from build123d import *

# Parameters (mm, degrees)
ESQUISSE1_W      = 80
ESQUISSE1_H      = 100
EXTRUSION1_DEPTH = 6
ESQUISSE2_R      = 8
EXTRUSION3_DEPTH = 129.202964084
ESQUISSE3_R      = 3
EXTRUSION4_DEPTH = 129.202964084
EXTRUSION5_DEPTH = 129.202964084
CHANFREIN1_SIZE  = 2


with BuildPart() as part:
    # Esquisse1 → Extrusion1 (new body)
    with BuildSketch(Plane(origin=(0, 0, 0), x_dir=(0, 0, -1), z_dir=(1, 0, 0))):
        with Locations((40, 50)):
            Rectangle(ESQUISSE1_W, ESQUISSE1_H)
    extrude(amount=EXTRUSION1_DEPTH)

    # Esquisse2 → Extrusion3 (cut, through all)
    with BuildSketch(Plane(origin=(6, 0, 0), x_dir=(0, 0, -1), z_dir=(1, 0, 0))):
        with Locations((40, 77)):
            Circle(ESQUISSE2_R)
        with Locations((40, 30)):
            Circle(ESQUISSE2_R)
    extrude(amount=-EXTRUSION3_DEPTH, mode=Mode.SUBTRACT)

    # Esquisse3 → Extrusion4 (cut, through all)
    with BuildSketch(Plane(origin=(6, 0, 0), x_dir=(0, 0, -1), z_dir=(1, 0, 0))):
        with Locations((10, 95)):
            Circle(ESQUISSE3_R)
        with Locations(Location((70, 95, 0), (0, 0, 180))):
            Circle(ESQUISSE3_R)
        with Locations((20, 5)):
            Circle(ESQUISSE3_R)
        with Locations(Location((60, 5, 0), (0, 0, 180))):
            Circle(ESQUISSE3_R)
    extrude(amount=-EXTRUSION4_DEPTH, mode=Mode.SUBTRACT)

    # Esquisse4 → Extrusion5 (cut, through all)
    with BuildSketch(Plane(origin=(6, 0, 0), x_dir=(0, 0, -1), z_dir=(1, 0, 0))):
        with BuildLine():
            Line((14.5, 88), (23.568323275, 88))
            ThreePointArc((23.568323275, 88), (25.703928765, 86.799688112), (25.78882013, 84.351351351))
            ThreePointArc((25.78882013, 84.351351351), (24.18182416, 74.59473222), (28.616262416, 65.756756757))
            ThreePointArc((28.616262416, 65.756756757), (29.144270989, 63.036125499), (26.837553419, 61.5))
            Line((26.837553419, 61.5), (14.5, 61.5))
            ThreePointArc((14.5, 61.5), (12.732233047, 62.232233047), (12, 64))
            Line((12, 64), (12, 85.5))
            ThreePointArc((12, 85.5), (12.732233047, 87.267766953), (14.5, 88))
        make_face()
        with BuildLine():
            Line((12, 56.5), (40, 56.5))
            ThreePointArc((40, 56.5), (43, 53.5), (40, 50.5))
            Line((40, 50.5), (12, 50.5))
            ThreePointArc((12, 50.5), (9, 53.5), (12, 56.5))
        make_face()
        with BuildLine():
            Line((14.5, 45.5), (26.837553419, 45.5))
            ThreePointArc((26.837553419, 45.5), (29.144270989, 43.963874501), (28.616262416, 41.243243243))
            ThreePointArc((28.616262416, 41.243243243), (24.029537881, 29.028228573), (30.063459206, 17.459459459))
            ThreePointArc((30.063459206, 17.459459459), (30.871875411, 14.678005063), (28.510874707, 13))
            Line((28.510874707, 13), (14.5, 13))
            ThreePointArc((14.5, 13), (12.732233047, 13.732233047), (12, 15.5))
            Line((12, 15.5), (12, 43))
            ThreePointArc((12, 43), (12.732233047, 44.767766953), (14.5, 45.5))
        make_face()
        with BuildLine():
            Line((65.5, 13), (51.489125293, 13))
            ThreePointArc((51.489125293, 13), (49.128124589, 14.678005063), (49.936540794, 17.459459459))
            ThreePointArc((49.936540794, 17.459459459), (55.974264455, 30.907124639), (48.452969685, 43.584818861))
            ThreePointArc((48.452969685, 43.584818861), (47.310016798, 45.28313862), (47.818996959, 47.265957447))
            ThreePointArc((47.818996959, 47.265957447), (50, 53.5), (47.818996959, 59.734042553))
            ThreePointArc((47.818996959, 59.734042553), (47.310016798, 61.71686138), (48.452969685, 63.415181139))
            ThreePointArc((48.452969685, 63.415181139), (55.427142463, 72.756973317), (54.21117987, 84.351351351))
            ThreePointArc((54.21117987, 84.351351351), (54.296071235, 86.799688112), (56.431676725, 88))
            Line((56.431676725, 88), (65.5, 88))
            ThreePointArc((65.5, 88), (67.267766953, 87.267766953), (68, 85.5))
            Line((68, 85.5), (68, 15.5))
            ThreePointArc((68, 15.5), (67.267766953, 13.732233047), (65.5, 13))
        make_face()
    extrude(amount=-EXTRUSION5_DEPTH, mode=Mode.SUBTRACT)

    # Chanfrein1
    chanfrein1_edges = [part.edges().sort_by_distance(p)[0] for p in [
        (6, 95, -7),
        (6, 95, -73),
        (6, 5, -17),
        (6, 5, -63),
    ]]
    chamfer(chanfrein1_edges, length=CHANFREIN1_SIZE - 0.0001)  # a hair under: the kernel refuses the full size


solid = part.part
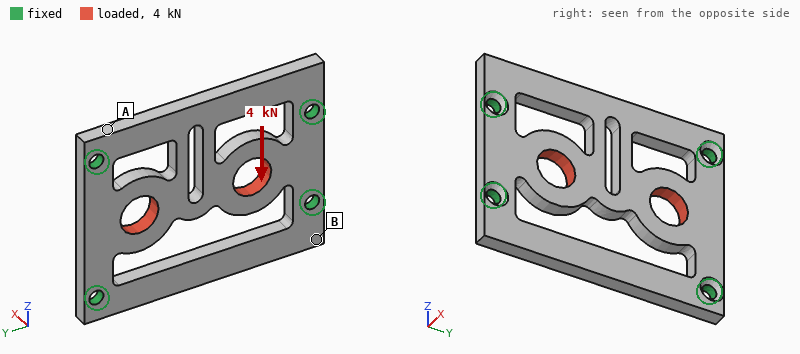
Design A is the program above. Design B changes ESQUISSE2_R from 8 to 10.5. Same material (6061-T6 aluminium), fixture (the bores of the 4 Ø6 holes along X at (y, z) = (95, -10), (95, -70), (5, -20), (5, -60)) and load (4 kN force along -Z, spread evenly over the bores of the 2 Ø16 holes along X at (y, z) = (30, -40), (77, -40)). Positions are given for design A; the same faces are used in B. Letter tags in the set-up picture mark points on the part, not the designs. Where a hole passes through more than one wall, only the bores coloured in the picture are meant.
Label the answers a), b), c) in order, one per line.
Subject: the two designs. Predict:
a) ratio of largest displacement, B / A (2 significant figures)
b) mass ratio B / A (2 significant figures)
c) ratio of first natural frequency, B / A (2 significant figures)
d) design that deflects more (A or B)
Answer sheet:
a) 1.5
b) 0.94
c) 1.0
d) B
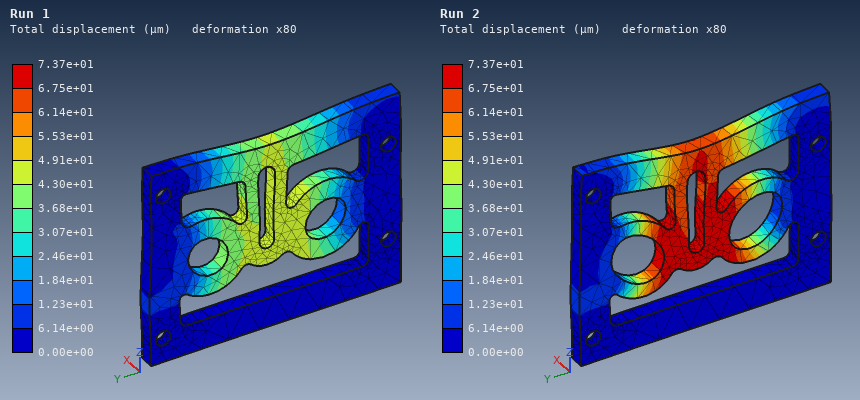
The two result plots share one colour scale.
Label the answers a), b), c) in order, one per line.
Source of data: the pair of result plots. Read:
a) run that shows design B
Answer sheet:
a) Run 2
